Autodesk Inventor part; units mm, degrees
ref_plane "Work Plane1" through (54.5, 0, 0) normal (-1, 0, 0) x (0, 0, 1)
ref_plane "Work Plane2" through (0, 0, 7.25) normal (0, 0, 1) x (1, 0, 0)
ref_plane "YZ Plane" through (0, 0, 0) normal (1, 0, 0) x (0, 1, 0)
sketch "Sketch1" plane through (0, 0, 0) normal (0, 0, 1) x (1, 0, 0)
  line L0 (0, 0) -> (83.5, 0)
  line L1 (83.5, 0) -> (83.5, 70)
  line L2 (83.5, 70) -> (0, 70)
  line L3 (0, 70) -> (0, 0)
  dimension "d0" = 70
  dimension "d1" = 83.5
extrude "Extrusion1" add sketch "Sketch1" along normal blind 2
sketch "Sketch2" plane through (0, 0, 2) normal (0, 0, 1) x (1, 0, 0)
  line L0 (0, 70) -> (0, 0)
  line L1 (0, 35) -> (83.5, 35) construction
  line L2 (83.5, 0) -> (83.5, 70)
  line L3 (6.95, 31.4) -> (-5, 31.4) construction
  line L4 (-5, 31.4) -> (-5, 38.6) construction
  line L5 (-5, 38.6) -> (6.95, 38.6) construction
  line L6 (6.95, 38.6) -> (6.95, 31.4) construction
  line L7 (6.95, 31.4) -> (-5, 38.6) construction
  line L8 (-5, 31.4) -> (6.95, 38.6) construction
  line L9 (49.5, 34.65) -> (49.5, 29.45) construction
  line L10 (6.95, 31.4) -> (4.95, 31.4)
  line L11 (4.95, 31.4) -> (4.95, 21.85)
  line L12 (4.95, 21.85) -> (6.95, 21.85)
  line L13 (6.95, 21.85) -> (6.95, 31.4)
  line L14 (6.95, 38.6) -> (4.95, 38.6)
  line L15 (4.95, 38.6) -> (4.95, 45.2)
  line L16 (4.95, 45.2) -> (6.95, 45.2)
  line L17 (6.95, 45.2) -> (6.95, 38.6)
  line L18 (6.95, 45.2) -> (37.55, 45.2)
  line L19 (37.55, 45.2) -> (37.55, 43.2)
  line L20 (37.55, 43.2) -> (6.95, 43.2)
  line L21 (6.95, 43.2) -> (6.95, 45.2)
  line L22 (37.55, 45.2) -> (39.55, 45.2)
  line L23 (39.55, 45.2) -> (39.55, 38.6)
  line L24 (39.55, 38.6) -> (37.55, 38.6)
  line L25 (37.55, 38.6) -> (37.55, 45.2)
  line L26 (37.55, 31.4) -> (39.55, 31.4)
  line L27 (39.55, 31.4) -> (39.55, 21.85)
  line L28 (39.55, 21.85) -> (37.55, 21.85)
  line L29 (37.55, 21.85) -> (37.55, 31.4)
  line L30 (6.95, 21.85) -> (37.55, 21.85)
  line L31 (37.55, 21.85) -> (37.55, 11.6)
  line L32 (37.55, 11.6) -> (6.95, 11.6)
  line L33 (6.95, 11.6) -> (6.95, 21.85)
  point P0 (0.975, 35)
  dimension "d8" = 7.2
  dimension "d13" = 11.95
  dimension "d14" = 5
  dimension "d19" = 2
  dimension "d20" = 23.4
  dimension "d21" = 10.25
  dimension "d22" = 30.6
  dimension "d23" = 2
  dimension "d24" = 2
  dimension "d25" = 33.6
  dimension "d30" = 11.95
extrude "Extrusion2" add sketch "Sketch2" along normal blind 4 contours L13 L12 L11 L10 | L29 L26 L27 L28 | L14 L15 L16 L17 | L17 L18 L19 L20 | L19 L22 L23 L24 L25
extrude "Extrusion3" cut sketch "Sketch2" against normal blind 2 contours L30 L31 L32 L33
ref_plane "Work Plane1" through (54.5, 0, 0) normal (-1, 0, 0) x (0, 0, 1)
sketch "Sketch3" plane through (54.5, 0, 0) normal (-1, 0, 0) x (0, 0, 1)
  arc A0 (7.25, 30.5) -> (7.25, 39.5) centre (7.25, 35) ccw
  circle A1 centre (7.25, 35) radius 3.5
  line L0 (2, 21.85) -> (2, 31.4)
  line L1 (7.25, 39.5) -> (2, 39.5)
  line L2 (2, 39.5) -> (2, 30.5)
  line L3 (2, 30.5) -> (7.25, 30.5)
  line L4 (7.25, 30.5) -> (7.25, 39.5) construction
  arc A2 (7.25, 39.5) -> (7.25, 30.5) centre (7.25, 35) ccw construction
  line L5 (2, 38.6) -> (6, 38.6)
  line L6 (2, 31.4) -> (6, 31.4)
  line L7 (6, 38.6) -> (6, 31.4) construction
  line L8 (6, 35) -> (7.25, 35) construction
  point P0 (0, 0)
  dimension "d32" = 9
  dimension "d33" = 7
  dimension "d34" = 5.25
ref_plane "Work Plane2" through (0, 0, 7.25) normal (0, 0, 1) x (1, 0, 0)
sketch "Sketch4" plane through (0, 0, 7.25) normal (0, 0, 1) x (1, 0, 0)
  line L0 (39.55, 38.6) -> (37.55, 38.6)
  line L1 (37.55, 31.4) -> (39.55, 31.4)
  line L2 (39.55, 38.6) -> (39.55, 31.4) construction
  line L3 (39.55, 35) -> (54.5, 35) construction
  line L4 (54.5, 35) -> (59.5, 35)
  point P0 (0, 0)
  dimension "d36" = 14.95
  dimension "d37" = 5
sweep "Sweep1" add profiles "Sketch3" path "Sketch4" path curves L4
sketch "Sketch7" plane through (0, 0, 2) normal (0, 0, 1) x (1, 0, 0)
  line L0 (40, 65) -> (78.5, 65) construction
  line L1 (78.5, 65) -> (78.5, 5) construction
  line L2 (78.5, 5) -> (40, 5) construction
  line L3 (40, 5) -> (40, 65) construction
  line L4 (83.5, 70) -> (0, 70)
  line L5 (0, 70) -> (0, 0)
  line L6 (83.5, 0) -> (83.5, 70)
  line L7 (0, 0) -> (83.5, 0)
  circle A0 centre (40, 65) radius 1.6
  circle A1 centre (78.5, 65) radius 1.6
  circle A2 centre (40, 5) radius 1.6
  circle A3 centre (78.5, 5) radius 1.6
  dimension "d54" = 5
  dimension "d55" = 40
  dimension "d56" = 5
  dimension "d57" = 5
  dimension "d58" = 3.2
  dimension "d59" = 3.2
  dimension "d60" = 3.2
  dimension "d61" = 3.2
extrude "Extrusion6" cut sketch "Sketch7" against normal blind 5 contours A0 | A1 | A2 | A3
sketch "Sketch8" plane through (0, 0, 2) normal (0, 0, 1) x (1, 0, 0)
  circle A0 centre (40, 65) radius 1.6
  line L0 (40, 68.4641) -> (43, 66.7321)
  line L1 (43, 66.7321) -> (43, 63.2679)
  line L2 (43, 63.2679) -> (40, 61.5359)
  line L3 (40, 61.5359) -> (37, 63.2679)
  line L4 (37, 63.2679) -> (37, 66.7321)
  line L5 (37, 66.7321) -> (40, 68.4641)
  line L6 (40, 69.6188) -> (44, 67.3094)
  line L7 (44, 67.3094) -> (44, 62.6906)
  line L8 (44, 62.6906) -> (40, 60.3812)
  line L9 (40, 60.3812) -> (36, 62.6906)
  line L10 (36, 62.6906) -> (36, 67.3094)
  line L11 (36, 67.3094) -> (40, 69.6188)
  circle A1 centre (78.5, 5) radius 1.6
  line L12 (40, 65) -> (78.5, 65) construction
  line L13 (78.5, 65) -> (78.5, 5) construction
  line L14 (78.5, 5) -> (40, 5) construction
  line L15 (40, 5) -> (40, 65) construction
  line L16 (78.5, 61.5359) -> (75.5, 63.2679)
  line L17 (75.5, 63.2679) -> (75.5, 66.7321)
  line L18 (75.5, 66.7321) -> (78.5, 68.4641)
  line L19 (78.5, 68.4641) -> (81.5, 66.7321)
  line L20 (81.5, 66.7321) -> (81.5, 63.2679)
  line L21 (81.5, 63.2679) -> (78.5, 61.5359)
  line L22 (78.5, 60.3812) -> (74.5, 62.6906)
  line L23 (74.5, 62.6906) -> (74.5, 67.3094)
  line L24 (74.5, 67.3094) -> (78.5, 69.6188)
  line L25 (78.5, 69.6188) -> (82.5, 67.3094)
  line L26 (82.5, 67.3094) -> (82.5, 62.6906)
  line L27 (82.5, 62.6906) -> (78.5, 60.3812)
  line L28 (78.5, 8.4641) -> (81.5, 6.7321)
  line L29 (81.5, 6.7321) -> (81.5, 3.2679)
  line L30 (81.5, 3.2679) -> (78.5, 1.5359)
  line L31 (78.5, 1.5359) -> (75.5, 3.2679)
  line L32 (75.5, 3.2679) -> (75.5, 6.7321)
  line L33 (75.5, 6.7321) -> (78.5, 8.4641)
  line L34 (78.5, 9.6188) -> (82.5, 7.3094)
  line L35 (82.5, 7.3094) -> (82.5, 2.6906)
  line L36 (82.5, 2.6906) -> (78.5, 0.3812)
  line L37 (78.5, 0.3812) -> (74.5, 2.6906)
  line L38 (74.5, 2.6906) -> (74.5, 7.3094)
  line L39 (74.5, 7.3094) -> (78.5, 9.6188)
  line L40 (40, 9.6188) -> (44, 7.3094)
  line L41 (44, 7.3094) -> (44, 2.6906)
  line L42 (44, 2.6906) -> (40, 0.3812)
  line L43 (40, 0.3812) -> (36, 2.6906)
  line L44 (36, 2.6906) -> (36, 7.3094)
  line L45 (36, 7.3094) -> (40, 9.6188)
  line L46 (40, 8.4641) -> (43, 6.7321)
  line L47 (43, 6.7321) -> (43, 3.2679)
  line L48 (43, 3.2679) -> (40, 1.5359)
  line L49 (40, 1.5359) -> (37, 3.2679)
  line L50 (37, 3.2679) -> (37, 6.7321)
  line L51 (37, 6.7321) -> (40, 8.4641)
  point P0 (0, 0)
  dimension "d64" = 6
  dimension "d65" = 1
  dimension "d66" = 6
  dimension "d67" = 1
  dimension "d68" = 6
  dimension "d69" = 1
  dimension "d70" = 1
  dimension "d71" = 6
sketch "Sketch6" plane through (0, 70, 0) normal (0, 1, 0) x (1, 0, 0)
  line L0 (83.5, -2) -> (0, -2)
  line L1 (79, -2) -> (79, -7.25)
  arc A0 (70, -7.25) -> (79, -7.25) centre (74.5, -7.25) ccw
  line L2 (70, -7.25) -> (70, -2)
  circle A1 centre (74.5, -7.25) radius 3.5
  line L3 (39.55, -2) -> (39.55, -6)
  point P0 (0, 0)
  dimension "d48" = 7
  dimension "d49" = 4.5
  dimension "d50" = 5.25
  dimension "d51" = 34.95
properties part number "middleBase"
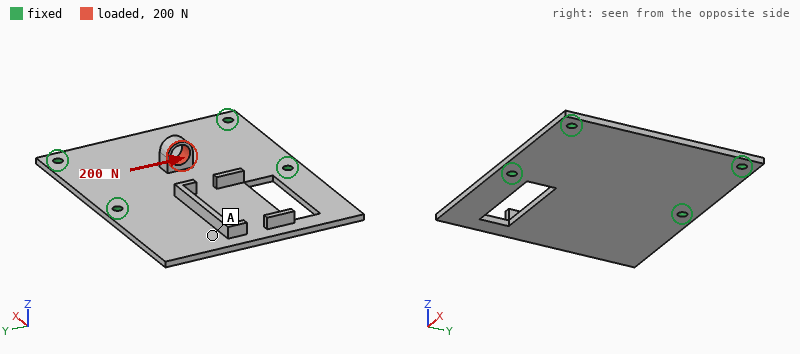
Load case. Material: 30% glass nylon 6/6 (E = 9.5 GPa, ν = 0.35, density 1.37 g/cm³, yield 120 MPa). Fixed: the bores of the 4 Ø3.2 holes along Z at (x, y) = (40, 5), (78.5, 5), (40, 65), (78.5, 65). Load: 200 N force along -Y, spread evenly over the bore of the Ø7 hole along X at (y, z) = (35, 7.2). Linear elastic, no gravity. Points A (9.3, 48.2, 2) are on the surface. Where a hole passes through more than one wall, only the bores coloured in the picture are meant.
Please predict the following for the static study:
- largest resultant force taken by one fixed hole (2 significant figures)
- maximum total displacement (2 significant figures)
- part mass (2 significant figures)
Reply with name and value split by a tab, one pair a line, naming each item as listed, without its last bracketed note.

largest resultant force taken by one fixed hole	63 N
maximum total displacement	0.36 mm
part mass	16 g
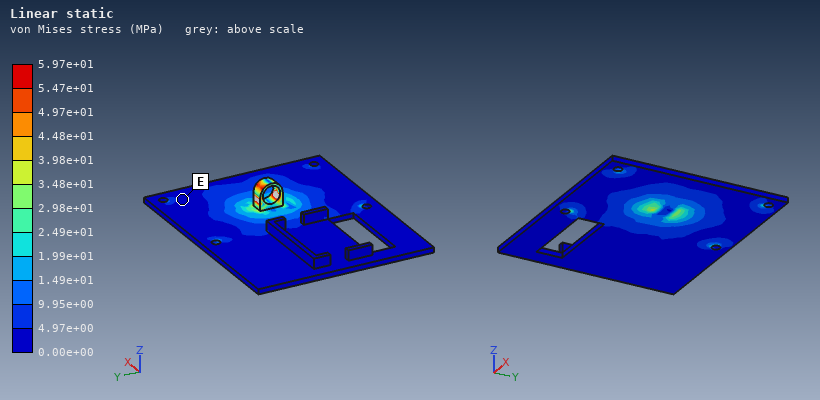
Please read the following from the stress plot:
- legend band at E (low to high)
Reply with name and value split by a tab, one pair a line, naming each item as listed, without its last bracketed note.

legend band at E	0.00e+00 to 4.97e+00 MPa
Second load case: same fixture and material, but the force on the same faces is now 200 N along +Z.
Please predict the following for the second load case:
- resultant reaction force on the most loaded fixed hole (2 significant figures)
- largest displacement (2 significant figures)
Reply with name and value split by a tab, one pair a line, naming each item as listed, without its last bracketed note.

resultant reaction force on the most loaded fixed hole	59 N
largest displacement	0.89 mm
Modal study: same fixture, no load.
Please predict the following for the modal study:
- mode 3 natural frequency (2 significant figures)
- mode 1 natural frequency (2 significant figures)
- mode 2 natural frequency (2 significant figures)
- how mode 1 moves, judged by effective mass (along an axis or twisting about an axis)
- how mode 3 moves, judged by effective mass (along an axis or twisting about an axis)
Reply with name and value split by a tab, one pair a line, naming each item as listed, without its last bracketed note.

mode 3 natural frequency	1300 Hz
mode 1 natural frequency	450 Hz
mode 2 natural frequency	880 Hz
how mode 1 moves, judged by effective mass	along Z
how mode 3 moves, judged by effective mass	along Z
